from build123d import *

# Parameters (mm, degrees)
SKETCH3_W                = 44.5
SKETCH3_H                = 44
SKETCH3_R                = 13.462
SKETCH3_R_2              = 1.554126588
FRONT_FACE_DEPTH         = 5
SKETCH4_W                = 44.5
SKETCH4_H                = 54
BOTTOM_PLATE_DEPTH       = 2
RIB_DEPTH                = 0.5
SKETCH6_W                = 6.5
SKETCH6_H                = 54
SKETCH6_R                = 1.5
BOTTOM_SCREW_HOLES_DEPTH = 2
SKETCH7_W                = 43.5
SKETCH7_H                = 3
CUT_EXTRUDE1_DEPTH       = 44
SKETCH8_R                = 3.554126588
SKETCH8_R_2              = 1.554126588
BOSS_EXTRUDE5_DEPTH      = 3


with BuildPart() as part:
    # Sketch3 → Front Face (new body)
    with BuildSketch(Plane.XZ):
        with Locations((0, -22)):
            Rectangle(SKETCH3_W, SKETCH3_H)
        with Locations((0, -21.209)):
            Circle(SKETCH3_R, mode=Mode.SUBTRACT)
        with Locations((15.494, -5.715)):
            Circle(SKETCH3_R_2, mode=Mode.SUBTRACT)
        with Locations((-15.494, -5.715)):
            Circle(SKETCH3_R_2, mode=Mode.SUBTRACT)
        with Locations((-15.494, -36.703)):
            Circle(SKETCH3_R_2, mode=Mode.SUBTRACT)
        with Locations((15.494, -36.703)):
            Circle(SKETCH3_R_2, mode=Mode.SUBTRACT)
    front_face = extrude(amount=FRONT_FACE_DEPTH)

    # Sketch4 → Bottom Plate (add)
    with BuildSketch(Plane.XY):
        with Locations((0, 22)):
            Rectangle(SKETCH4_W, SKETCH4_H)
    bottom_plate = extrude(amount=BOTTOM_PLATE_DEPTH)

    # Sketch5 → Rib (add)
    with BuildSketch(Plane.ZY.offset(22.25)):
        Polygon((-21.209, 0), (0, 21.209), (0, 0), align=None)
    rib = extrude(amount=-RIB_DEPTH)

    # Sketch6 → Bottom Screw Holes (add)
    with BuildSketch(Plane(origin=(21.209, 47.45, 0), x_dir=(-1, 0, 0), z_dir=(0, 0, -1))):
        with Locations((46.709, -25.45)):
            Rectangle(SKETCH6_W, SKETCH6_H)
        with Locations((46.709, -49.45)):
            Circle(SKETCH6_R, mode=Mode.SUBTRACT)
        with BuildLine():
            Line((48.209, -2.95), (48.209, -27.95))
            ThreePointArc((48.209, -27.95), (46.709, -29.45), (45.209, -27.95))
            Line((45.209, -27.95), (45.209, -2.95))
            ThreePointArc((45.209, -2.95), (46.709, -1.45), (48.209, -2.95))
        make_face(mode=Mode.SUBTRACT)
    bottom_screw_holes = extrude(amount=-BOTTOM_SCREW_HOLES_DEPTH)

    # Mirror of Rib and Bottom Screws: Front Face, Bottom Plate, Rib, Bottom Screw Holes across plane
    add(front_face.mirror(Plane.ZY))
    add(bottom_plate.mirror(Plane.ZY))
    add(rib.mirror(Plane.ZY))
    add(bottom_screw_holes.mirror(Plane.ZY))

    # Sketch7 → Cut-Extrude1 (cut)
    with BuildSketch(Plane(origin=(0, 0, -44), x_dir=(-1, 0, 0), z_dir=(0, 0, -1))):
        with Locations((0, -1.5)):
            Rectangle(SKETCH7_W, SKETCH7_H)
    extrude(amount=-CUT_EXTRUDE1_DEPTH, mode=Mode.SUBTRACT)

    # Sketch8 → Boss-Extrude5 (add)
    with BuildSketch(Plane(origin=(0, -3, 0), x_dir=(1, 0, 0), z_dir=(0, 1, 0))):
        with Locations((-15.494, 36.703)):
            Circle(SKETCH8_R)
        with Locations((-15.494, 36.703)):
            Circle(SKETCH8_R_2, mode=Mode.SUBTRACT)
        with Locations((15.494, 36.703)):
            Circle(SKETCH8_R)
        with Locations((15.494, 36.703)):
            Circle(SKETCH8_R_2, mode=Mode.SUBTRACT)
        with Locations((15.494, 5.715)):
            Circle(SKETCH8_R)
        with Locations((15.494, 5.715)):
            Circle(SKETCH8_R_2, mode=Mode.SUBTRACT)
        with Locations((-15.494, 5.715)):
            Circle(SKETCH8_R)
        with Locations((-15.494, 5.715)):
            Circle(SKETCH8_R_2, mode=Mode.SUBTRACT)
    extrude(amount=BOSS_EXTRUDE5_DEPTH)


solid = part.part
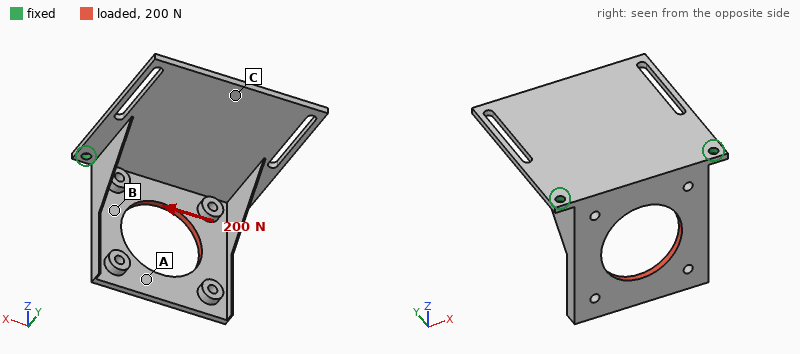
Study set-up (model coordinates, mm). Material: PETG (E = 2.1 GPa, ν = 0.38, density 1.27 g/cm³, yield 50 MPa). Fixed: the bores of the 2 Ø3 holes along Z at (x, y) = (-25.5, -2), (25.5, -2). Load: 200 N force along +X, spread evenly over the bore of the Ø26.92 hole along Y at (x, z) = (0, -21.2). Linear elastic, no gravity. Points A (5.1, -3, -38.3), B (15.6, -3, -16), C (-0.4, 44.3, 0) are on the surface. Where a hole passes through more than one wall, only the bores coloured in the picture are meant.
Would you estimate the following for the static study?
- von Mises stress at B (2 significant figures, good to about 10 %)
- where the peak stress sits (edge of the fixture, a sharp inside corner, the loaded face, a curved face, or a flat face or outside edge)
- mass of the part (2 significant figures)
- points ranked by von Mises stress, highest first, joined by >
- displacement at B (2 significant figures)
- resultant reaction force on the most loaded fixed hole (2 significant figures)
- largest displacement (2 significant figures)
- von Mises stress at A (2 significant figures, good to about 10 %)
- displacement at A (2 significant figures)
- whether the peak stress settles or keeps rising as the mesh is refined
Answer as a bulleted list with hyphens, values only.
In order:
- 9.1 MPa
- edge of the fixture
- 12 g
- B > A > C
- 0.32 mm
- 140 N
- 1.0 mm
- 3.9 MPa
- 0.63 mm
- keeps rising
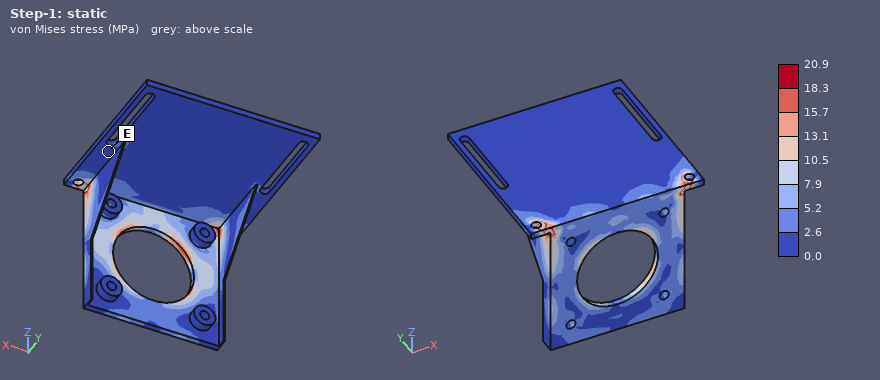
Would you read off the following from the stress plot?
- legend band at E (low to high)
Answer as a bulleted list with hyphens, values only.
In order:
- 0.0 to 2.6 MPa
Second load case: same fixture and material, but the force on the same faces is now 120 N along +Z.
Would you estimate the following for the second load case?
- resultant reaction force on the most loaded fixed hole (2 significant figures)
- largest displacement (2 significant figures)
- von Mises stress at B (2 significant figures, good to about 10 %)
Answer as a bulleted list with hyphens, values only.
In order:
- 68 N
- 0.98 mm
- 2.1 MPa
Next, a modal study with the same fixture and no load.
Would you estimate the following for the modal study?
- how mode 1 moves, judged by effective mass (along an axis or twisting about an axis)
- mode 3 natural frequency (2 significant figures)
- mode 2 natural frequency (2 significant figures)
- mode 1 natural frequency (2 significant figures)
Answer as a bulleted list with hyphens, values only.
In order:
- along Z
- 420 Hz
- 370 Hz
- 170 Hz
